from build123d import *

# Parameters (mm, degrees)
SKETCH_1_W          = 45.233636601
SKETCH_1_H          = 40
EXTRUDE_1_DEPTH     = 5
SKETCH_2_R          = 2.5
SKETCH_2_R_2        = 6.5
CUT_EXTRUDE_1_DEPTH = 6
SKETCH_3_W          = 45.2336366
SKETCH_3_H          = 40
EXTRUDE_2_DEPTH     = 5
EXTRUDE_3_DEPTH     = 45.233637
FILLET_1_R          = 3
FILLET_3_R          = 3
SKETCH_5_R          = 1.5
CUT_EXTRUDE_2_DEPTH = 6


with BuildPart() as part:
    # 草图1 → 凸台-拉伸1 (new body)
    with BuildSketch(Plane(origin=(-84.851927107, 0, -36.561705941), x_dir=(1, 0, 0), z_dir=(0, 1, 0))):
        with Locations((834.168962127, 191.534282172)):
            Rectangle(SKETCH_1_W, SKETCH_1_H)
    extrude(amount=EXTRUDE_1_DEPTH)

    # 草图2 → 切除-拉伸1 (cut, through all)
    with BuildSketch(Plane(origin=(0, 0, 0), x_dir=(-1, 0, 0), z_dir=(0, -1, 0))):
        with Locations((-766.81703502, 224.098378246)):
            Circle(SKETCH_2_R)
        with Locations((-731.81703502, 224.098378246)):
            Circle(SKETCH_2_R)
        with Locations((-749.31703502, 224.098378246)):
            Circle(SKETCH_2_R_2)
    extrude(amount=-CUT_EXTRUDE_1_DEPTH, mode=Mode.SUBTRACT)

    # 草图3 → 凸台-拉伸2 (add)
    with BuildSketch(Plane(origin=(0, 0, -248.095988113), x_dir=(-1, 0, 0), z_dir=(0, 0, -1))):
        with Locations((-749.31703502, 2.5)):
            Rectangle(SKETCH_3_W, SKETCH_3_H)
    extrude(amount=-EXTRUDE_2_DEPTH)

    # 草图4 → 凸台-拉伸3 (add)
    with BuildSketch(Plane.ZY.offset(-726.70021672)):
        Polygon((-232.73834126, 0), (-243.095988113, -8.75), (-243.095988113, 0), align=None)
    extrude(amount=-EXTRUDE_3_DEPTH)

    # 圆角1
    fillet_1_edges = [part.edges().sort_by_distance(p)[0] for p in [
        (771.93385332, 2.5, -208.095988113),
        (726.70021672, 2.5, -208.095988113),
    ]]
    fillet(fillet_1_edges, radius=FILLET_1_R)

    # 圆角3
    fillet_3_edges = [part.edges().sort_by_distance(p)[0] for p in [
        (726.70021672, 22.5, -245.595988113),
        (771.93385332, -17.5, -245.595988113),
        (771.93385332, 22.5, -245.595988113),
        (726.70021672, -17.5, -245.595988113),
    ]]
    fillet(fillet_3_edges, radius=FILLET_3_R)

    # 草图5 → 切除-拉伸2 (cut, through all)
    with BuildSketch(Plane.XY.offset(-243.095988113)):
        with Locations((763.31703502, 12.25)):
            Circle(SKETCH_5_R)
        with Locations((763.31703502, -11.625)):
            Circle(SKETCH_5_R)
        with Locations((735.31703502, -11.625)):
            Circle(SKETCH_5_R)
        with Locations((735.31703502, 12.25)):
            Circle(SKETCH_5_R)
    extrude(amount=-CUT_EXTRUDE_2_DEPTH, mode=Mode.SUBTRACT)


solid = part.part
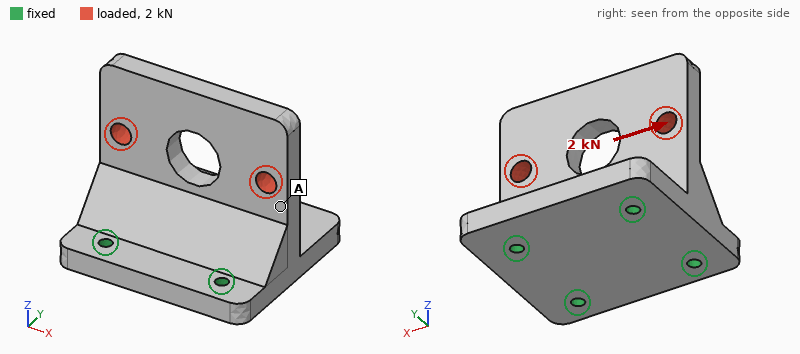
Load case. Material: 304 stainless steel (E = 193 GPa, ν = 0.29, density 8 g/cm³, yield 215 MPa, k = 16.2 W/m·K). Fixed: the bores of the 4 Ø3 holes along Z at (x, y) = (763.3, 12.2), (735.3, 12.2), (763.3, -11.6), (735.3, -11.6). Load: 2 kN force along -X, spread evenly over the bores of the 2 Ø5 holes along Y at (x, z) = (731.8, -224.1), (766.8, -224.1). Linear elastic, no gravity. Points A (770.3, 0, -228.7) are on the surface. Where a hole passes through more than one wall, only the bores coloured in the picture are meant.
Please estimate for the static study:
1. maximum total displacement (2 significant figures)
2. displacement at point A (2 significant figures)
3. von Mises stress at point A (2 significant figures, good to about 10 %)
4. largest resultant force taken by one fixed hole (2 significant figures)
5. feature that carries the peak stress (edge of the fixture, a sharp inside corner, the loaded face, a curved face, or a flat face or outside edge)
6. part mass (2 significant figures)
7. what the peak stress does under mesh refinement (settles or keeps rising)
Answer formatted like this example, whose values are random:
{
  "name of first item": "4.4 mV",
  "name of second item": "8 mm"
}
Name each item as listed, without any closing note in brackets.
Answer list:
{
  "maximum total displacement": "13 µm",
  "displacement at point A": "7.8 µm",
  "von Mises stress at point A": "11 MPa",
  "largest resultant force taken by one fixed hole": "1.1 kN",
  "feature that carries the peak stress": "edge of the fixture",
  "part mass": "140 g",
  "what the peak stress does under mesh refinement": "keeps rising"
}
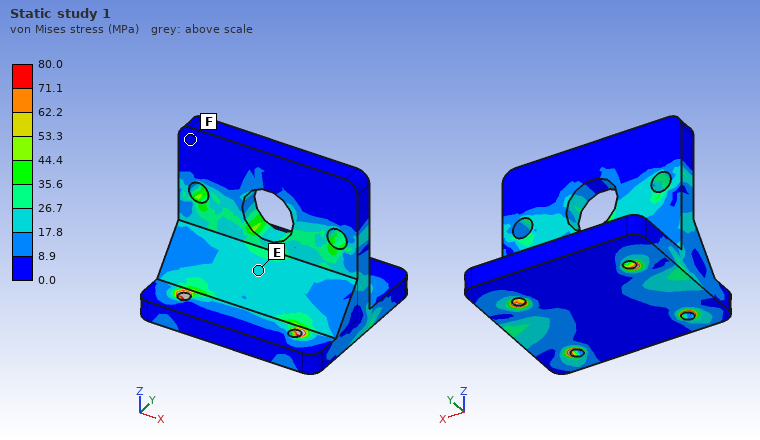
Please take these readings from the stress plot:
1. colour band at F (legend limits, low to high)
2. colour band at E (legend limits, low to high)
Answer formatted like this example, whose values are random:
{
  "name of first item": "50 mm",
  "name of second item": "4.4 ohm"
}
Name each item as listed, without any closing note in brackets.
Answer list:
{
  "colour band at F": "0.0 to 8.9 MPa",
  "colour band at E": "17.8 to 26.7 MPa"
}
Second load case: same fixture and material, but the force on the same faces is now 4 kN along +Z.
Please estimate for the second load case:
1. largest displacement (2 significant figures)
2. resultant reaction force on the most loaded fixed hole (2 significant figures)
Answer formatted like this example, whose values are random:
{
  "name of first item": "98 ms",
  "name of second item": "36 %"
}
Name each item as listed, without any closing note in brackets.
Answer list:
{
  "largest displacement": "14 µm",
  "resultant reaction force on the most loaded fixed hole": "1.3 kN"
}
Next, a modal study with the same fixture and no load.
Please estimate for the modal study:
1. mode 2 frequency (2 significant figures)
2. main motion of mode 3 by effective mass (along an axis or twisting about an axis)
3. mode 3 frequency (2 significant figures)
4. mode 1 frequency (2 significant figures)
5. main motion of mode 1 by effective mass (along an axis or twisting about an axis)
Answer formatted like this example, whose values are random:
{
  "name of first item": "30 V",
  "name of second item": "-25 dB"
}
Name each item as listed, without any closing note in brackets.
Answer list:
{
  "mode 2 frequency": "7200 Hz",
  "main motion of mode 3 by effective mass": "along X",
  "mode 3 frequency": "9600 Hz",
  "mode 1 frequency": "4100 Hz",
  "main motion of mode 1 by effective mass": "along Y"
}
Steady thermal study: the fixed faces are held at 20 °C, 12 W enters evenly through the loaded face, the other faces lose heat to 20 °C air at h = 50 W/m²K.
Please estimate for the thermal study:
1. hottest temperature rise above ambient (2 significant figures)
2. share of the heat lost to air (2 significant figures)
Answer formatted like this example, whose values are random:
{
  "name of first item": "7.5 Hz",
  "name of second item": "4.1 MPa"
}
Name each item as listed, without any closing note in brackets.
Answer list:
{
  "hottest temperature rise above ambient": "60 K",
  "share of the heat lost to air": "54 %"
}
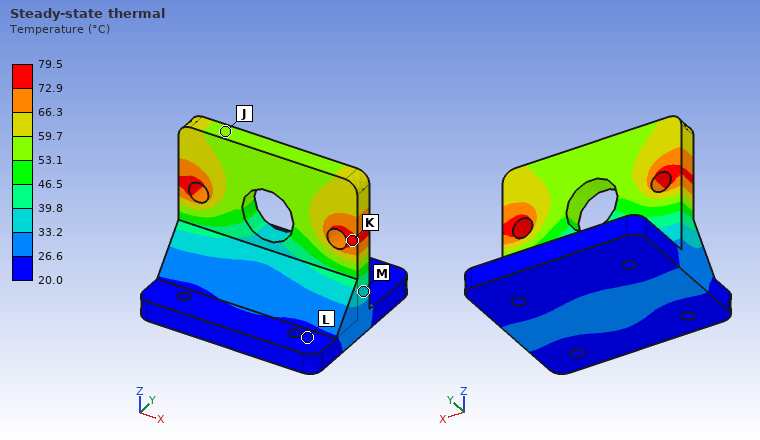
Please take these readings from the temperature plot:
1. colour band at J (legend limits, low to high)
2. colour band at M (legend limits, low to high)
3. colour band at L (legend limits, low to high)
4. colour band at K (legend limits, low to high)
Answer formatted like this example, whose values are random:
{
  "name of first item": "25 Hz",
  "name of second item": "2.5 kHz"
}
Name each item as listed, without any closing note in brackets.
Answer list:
{
  "colour band at J": "53.1 to 59.7 °C",
  "colour band at M": "33.2 to 39.8 °C",
  "colour band at L": "20.0 to 26.6 °C",
  "colour band at K": "72.9 to 79.5 °C"
}
